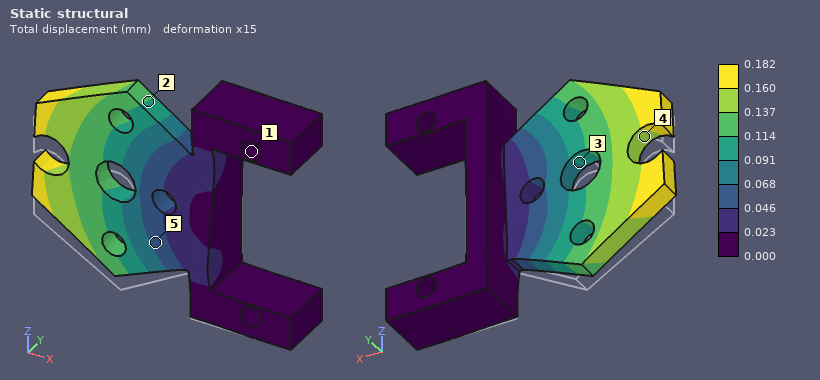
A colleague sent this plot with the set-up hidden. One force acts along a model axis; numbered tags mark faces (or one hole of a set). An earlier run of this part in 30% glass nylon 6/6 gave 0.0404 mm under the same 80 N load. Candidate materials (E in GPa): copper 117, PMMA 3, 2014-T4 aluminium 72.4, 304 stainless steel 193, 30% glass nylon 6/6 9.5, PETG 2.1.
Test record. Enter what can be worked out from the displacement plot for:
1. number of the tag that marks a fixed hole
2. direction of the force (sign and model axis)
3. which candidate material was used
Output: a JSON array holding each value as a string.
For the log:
["1", "+Z", "PETG"]
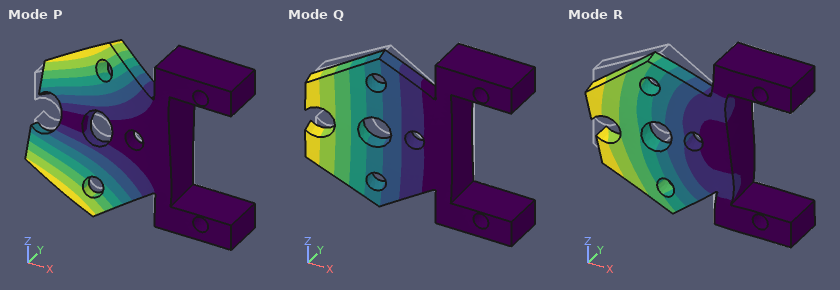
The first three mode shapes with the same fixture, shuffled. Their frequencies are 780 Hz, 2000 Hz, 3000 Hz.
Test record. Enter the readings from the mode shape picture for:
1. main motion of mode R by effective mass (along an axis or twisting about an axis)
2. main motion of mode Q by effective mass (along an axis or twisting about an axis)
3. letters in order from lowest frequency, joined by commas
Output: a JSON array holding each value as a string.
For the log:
["along Z", "along Y", "Q, P, R"]
